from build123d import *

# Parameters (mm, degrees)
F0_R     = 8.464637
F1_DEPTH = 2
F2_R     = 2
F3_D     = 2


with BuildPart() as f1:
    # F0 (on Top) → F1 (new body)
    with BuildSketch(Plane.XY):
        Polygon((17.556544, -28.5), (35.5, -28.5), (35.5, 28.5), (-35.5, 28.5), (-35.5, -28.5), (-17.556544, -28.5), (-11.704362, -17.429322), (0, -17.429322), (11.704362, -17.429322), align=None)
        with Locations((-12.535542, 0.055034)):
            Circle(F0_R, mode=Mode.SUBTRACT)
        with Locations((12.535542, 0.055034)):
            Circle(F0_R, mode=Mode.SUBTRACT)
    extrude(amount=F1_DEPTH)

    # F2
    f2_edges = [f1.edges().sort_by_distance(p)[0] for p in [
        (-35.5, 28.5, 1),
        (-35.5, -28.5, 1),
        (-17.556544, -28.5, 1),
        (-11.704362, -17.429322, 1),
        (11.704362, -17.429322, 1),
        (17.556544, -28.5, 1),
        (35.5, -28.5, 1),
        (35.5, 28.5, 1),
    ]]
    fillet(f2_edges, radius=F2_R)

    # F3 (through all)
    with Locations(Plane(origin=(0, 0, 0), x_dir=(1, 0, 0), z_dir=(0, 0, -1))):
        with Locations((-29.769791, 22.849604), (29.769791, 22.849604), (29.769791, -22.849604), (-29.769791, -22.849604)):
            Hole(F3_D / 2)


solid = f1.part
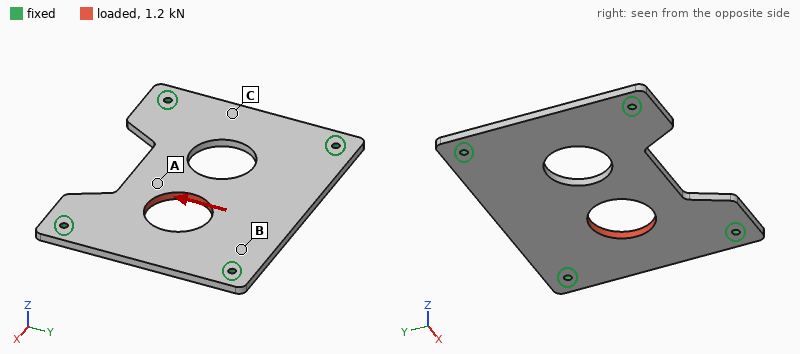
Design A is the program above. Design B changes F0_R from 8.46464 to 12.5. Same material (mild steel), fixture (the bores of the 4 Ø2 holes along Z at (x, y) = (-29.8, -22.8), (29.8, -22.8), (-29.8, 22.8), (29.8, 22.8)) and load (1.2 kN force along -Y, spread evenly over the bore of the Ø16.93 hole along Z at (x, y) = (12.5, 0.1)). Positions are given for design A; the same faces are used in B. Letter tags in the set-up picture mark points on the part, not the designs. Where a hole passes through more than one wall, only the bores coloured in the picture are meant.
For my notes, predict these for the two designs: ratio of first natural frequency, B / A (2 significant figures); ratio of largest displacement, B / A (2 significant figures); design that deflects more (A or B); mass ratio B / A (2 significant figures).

1.1
2.0
B
0.84
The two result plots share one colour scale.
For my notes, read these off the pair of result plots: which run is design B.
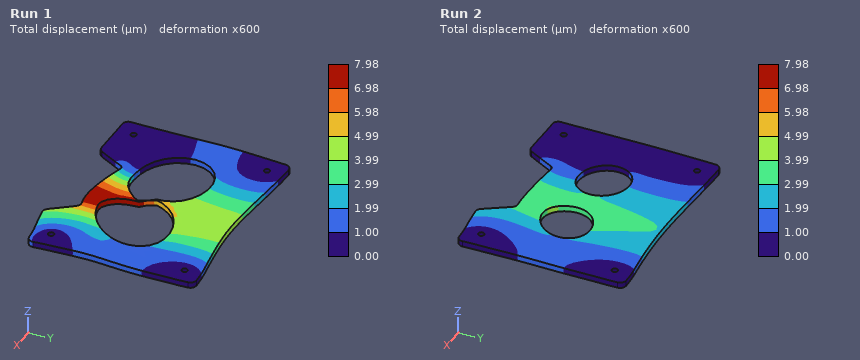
Run 1
